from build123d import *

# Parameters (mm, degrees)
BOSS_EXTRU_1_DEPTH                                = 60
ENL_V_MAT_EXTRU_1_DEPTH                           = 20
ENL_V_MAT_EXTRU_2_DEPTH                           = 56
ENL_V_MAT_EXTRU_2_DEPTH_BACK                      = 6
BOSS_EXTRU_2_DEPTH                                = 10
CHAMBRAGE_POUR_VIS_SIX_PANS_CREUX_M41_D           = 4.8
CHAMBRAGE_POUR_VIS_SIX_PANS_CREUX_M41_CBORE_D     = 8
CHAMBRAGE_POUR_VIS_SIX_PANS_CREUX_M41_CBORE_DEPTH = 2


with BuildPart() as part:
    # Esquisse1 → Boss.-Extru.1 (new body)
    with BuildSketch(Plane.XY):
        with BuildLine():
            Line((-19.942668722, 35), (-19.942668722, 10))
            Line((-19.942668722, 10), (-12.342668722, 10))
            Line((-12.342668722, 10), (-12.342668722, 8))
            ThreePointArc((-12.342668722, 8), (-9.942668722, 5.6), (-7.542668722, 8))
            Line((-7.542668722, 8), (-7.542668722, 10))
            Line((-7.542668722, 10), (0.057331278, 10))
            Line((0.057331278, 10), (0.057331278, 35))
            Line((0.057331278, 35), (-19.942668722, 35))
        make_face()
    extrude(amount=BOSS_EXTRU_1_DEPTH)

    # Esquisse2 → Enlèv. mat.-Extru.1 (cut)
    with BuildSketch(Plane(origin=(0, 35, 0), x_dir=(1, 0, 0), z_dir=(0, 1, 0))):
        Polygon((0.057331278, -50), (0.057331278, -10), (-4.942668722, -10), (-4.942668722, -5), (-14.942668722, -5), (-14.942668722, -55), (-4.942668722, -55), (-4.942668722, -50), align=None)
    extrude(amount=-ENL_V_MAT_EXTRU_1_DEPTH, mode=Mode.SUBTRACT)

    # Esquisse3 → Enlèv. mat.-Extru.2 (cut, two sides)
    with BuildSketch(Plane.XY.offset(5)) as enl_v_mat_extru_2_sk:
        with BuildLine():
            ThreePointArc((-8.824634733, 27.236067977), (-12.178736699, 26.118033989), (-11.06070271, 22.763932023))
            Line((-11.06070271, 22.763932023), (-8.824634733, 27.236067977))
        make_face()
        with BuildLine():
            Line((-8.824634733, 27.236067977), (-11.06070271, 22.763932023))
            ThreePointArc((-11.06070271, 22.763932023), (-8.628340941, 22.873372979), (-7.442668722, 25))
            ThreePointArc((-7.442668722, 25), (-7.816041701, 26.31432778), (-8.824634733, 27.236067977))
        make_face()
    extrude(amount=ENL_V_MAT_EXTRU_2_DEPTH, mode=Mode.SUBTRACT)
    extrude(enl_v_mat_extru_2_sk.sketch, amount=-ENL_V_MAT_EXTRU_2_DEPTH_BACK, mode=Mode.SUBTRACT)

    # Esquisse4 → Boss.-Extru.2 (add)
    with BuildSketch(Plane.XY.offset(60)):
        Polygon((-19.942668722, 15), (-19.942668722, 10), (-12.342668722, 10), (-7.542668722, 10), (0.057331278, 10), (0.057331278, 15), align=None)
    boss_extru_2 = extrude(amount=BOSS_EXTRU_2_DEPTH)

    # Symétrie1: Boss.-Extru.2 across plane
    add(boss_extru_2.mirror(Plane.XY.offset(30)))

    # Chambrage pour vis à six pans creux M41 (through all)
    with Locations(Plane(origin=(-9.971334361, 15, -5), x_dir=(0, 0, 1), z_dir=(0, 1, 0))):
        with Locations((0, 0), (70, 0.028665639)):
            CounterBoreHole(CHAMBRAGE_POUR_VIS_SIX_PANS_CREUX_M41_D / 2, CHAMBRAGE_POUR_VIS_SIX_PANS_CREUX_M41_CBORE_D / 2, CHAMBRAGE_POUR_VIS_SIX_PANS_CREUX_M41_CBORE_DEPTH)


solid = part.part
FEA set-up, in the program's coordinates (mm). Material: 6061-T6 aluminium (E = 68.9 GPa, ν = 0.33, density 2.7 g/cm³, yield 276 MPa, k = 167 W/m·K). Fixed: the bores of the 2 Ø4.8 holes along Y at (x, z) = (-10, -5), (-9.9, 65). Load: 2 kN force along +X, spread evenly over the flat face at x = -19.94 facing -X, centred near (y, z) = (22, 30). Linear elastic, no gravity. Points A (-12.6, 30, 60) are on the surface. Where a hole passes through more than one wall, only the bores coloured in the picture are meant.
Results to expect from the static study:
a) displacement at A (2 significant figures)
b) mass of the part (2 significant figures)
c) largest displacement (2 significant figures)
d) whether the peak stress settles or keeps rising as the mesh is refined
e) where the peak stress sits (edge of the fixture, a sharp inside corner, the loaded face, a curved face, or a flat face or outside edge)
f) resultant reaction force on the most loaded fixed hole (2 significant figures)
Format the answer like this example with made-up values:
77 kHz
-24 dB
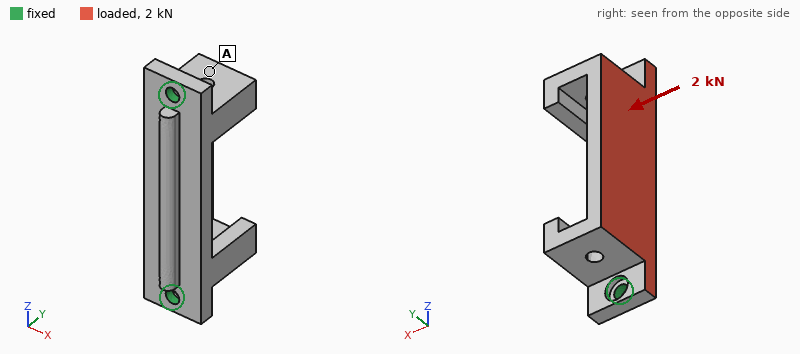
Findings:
0.11 mm
50 g
0.19 mm
keeps rising
edge of the fixture
1.0 kN
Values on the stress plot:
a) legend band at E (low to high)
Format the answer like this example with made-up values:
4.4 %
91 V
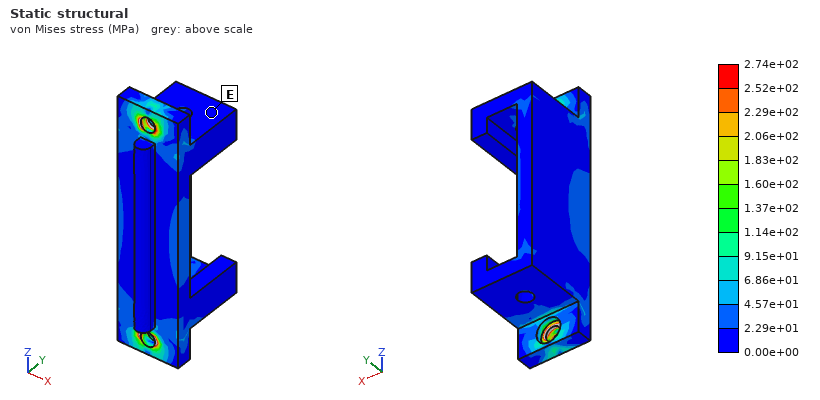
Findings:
0.00e+00 to 2.29e+01 MPa
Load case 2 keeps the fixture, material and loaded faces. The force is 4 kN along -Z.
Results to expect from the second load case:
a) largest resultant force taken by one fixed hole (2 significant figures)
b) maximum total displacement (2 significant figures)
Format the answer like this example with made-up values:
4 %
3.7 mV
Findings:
2.2 kN
19 µm
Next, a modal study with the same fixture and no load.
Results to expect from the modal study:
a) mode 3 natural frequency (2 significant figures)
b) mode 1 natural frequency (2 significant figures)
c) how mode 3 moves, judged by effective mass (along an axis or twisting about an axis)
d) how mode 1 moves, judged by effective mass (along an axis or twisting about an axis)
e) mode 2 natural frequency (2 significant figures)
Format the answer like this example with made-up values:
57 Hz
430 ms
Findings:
7200 Hz
3400 Hz
along Y
along X
6500 Hz
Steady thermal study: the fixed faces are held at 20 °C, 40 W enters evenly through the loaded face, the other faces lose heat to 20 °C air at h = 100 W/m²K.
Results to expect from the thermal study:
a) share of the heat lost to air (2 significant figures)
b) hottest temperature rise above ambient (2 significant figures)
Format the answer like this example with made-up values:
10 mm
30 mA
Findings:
21 %
19 K
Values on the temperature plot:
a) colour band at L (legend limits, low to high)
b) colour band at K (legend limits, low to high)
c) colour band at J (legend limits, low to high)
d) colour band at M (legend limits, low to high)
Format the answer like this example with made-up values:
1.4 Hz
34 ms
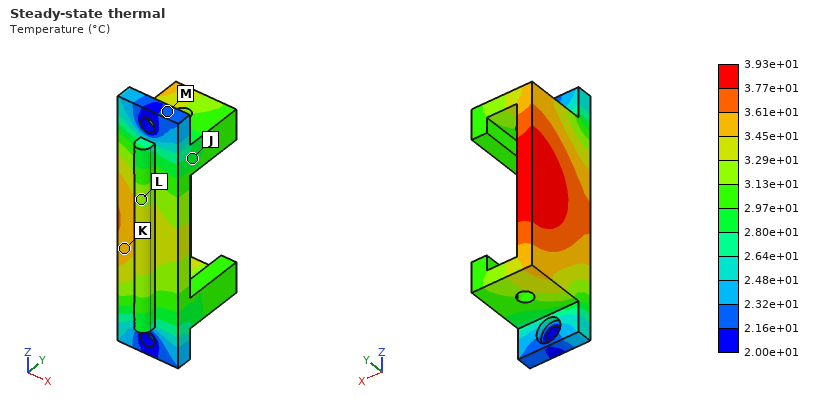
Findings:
3.13e+01 to 3.29e+01 °C
3.45e+01 to 3.61e+01 °C
2.80e+01 to 2.97e+01 °C
2.16e+01 to 2.32e+01 °C
